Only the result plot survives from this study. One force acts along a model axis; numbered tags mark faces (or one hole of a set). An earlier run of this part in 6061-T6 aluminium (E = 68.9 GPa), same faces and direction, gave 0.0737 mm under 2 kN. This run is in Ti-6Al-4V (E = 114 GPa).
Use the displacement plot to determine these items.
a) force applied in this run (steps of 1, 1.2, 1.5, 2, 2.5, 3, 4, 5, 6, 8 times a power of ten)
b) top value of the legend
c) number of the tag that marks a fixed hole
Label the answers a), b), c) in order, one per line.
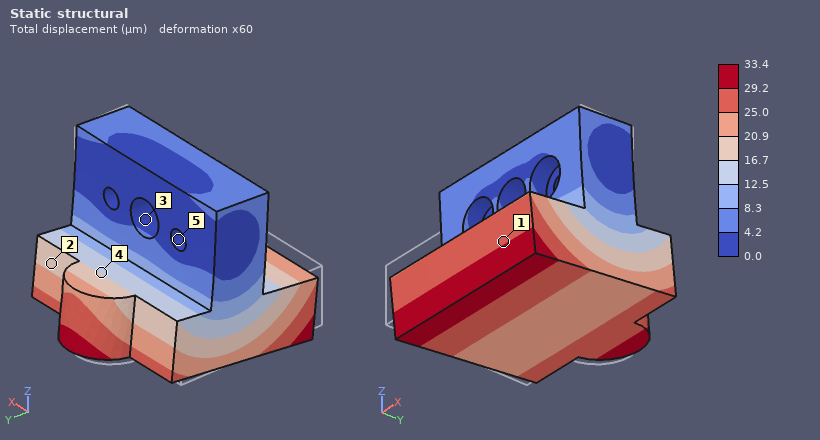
a) 1.5 kN
b) 33.4 µm
c) 5
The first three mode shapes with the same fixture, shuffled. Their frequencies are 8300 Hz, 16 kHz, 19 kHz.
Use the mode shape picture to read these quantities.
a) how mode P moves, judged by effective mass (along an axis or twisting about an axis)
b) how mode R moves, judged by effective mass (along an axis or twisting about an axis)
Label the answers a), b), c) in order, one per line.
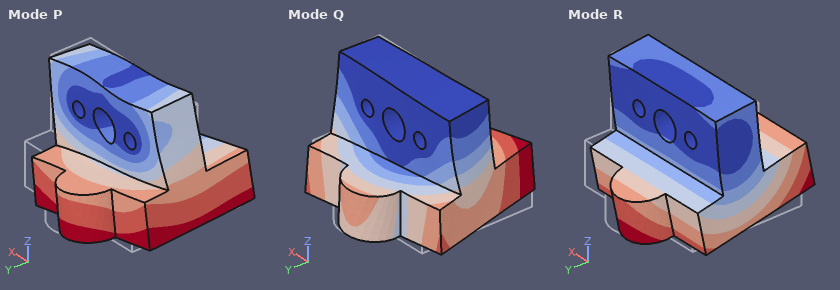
a) along X
b) along Y
